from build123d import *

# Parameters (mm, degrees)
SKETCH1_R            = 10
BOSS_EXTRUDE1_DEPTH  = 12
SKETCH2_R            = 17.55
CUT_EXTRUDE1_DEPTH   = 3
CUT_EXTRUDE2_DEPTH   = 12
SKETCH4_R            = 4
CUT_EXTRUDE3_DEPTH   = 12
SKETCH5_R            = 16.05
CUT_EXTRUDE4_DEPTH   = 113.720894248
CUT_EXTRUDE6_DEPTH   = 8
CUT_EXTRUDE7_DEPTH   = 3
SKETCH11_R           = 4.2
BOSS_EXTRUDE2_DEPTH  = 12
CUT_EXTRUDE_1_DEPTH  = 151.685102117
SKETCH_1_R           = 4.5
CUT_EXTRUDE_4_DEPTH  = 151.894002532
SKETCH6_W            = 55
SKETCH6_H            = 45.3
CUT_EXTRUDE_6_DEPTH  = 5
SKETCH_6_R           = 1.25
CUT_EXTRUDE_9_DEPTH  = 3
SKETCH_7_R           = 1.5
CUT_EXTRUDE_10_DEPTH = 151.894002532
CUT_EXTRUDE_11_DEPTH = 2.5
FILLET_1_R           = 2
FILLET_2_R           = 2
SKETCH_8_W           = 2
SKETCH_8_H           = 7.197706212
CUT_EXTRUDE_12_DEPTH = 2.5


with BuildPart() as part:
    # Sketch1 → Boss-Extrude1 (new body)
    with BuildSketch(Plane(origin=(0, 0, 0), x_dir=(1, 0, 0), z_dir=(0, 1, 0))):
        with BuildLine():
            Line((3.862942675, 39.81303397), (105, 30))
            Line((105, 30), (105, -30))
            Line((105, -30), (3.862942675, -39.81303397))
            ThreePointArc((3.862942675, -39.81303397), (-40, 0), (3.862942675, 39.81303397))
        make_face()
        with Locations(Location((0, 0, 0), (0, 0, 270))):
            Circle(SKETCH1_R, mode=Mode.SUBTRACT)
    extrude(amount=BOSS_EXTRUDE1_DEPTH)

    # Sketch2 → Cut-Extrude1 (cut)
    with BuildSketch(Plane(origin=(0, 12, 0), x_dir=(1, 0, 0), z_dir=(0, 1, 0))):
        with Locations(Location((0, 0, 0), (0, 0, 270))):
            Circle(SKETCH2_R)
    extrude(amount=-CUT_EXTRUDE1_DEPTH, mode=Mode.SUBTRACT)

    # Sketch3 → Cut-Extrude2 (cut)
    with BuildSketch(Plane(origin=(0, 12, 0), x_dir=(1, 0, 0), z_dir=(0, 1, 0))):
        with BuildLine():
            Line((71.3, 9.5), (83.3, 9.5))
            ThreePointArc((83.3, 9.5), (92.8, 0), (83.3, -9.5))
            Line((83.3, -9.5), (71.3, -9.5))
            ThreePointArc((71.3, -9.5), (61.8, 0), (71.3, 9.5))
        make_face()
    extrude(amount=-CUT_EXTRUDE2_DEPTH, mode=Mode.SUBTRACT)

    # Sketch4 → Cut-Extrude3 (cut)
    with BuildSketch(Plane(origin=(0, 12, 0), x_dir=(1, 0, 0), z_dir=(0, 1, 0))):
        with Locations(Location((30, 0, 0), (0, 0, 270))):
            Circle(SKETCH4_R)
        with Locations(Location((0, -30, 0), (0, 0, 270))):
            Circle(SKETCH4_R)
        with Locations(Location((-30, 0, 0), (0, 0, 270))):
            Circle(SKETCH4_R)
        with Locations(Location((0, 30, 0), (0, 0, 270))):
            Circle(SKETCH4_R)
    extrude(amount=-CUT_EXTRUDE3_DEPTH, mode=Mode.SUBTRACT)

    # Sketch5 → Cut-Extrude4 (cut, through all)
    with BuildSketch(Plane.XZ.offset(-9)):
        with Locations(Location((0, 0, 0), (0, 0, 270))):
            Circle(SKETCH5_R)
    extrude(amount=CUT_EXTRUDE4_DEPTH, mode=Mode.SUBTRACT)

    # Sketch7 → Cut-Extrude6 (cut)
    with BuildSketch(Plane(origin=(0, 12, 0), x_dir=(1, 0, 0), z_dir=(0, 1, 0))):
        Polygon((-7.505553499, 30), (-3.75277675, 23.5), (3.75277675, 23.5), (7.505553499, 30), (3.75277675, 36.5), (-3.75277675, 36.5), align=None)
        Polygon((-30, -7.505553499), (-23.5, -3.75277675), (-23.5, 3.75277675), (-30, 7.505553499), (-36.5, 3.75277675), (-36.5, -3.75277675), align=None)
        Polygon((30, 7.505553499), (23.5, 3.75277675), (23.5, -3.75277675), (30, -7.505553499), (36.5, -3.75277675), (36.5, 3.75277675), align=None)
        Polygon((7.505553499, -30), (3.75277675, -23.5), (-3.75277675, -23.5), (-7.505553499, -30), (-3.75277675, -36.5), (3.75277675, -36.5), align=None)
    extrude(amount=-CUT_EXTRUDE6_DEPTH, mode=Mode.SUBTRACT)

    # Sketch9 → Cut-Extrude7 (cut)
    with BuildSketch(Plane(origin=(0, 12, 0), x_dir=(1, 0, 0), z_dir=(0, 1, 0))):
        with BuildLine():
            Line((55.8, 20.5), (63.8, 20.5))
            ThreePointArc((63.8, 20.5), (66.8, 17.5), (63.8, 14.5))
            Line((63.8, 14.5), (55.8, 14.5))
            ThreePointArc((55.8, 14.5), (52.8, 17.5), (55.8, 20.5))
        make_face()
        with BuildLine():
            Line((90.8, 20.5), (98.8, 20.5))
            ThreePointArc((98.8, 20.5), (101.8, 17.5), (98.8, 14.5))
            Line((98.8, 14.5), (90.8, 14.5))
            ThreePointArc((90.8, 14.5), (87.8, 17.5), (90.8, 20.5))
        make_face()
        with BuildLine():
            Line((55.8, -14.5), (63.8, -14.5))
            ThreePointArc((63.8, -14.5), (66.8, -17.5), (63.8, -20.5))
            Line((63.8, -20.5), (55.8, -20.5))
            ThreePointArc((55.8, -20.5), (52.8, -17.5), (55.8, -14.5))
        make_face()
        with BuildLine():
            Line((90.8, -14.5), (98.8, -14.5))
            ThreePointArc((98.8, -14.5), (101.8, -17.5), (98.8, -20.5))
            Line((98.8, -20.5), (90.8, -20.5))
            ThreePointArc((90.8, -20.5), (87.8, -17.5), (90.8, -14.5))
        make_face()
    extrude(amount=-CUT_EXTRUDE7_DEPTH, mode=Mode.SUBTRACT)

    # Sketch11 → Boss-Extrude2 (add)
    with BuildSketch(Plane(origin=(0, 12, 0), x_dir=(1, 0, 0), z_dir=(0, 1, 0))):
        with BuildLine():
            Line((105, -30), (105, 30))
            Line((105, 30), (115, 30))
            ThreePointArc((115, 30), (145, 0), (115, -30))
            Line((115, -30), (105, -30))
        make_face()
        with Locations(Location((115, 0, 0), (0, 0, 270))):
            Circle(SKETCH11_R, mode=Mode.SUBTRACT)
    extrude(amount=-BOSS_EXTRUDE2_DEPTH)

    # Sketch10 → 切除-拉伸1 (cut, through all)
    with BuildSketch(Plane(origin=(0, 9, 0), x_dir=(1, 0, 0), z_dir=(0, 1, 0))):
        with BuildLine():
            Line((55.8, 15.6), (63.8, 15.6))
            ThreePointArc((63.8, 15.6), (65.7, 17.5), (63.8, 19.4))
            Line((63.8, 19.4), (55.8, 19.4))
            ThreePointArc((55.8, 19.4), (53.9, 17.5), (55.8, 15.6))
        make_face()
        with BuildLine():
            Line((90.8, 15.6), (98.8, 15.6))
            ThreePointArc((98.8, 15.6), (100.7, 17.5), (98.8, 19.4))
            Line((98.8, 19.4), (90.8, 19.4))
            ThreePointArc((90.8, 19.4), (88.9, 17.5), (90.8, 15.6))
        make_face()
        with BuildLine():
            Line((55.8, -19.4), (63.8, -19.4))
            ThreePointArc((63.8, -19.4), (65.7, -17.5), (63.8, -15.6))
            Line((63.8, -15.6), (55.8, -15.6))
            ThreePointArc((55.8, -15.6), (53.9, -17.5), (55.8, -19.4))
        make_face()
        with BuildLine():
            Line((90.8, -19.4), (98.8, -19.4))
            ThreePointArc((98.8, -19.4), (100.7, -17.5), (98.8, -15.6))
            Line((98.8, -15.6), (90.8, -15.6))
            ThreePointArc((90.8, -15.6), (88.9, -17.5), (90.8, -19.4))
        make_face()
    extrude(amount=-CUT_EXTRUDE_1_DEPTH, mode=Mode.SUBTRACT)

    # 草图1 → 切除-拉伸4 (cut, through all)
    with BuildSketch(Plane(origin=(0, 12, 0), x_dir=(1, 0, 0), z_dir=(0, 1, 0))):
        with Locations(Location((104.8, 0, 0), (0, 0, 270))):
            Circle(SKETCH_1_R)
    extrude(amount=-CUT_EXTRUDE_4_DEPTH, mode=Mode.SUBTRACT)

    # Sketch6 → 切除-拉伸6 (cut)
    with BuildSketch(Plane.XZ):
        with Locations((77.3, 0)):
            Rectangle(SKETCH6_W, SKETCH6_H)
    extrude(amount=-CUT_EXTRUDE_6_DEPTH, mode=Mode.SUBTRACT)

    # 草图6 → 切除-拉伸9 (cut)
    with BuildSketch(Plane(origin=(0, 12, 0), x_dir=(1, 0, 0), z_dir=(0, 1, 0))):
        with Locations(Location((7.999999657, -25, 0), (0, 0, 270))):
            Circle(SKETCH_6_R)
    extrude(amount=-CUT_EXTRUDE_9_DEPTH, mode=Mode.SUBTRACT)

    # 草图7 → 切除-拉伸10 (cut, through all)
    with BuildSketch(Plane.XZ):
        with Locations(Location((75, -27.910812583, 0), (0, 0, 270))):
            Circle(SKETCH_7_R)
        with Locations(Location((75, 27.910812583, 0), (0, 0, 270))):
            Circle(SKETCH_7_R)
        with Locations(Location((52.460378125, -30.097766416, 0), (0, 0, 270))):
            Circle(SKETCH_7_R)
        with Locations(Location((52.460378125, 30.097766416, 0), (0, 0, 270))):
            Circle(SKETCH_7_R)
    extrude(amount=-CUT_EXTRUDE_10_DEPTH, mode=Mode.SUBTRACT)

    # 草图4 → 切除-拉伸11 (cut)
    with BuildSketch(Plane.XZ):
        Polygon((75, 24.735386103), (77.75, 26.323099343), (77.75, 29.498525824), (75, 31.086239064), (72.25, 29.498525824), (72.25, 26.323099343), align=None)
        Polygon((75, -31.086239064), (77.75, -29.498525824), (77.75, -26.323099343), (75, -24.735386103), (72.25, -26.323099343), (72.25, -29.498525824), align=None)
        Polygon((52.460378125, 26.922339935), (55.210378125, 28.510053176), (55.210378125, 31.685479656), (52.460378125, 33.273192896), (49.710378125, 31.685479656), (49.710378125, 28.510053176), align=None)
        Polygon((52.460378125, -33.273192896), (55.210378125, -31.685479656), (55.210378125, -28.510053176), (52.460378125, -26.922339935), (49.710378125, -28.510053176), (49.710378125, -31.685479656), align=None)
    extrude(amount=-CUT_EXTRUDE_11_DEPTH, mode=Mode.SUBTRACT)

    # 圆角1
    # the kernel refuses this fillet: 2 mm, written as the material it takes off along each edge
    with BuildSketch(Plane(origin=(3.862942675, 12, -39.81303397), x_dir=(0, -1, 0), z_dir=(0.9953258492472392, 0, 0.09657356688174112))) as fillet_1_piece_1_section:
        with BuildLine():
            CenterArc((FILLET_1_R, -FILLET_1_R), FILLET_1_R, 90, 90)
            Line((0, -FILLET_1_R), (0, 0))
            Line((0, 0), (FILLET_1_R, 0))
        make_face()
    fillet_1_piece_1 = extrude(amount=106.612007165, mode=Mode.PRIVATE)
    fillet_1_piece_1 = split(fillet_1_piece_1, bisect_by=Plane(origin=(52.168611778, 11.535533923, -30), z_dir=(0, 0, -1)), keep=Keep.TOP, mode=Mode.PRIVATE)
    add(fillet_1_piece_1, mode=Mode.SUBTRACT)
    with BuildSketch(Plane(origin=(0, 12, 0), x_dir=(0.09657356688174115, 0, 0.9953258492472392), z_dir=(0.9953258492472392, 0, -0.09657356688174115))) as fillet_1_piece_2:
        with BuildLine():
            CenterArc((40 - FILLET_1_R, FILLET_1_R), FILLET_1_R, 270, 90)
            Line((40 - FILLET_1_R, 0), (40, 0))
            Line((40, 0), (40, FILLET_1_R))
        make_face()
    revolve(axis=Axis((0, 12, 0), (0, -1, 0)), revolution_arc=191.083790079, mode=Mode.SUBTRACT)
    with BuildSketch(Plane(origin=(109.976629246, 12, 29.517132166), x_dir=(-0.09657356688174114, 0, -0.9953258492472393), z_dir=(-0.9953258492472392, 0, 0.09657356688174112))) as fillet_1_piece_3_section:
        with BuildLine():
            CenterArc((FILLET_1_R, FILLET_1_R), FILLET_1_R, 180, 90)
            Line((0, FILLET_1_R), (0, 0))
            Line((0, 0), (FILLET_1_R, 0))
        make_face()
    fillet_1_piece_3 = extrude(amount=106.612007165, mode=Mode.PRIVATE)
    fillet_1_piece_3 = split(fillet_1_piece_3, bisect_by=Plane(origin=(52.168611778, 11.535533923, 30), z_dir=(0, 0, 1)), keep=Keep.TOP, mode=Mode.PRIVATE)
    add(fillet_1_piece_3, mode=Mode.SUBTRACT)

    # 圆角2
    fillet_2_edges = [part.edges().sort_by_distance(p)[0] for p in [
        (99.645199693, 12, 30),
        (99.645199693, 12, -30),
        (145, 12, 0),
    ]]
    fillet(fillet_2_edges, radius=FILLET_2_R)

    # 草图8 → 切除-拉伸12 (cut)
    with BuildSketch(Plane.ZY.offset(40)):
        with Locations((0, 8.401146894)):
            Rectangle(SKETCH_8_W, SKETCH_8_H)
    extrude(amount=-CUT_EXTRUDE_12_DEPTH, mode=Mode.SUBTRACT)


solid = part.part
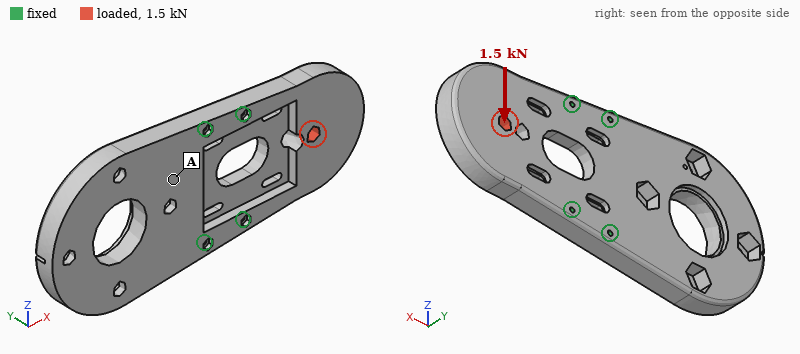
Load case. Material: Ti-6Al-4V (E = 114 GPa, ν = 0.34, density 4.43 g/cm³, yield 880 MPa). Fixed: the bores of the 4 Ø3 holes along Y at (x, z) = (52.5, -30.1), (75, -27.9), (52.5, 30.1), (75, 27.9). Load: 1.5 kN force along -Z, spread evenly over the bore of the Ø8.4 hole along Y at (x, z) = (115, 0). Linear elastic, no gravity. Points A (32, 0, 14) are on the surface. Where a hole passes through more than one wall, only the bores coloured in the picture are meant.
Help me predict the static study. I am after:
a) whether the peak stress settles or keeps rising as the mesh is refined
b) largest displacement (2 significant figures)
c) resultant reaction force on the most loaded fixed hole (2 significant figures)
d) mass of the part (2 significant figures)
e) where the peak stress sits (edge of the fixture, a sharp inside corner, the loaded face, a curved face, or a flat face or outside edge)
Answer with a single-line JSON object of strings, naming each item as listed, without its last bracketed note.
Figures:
{"whether the peak stress settles or keeps rising as the mesh is refined": "keeps rising", "largest displacement": "10 µm", "resultant reaction force on the most loaded fixed hole": "1.2 kN", "mass of the part": "480 g", "where the peak stress sits": "edge of the fixture"}
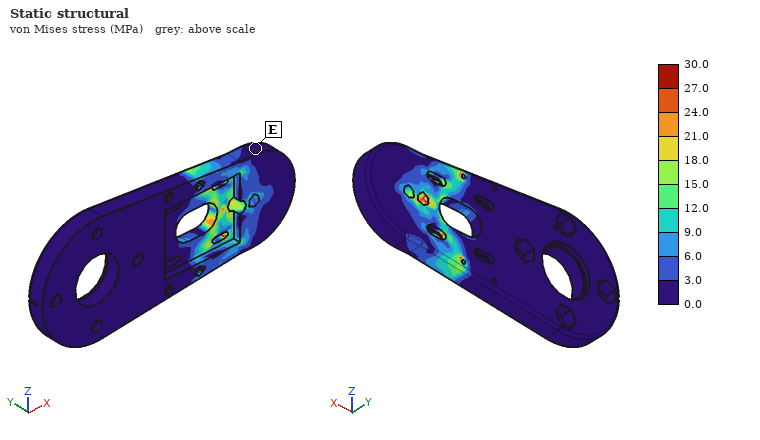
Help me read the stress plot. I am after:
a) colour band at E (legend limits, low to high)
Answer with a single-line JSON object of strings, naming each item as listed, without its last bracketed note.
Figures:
{"colour band at E": "0.0 to 3.0 MPa"}
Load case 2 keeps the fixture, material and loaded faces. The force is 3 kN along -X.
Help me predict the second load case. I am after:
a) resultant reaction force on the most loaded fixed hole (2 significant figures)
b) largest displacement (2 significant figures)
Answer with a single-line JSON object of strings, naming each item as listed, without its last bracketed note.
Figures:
{"resultant reaction force on the most loaded fixed hole": "1.2 kN", "largest displacement": "20 µm"}
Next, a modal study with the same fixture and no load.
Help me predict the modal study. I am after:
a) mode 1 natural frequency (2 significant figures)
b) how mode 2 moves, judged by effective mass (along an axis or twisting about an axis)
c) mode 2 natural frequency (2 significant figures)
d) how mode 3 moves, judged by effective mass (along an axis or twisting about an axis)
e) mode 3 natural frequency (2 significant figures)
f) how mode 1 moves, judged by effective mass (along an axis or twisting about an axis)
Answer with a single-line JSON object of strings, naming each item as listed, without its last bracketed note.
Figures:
{"mode 1 natural frequency": "1000 Hz", "how mode 2 moves, judged by effective mass": "along Y", "mode 2 natural frequency": "1400 Hz", "how mode 3 moves, judged by effective mass": "twisting about X", "mode 3 natural frequency": "3000 Hz", "how mode 1 moves, judged by effective mass": "along Y"}
